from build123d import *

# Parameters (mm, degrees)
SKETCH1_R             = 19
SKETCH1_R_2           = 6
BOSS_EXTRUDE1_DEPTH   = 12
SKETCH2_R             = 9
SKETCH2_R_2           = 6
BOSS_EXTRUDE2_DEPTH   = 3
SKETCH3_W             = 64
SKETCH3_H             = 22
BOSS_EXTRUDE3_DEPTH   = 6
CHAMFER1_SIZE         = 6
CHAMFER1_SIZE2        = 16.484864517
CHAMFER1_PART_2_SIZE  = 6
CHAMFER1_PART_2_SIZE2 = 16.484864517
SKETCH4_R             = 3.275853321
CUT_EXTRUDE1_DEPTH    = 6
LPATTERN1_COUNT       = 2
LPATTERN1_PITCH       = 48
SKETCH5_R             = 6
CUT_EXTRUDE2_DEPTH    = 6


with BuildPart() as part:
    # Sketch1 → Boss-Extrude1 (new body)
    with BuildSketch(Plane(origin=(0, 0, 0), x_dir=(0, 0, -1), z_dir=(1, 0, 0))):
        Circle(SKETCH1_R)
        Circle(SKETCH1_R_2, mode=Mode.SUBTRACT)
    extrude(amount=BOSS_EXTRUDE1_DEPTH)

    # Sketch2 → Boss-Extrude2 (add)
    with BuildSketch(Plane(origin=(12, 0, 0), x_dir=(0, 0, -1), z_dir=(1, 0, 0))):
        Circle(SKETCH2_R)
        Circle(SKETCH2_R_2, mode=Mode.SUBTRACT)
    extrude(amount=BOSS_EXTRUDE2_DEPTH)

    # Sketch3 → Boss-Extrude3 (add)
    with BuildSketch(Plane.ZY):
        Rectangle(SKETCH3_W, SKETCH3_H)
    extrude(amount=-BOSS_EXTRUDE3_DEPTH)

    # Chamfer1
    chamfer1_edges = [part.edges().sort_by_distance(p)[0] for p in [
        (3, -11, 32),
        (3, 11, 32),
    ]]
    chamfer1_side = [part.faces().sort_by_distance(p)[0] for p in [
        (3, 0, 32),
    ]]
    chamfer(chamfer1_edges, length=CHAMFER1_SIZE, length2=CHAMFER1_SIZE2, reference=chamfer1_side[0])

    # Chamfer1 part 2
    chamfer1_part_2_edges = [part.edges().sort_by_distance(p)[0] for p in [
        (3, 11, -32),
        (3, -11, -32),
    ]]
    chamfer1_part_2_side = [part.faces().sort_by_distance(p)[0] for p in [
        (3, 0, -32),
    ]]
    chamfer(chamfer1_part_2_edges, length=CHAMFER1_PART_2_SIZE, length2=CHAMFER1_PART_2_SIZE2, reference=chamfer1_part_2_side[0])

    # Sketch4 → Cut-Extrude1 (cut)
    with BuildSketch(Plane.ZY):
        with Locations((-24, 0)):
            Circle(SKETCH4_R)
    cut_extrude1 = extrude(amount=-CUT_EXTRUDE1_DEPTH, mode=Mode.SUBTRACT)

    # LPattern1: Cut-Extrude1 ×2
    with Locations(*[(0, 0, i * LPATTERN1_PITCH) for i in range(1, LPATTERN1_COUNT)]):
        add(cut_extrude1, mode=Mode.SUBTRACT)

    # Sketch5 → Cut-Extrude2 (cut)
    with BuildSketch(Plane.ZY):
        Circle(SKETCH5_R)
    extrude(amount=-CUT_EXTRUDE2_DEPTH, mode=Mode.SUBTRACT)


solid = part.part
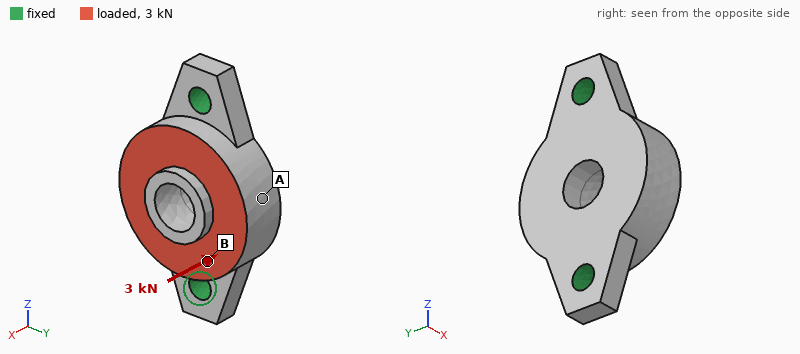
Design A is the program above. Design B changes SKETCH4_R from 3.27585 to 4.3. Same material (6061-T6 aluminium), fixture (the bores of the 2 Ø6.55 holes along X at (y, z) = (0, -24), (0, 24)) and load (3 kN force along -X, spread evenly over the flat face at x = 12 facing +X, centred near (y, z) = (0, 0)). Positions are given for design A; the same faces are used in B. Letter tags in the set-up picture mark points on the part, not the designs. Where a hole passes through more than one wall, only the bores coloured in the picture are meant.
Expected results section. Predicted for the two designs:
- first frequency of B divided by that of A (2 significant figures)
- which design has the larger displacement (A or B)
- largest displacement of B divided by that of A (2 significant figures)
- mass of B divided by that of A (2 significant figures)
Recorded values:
1.2
A
0.85
0.98
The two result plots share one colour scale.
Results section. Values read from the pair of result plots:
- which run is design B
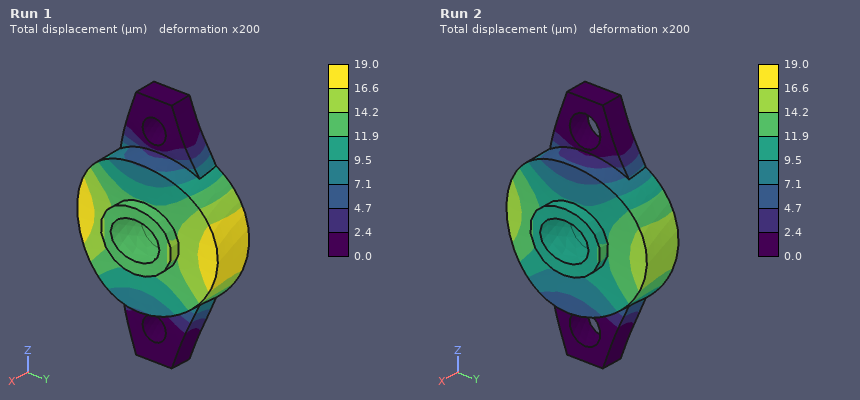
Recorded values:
Run 2
